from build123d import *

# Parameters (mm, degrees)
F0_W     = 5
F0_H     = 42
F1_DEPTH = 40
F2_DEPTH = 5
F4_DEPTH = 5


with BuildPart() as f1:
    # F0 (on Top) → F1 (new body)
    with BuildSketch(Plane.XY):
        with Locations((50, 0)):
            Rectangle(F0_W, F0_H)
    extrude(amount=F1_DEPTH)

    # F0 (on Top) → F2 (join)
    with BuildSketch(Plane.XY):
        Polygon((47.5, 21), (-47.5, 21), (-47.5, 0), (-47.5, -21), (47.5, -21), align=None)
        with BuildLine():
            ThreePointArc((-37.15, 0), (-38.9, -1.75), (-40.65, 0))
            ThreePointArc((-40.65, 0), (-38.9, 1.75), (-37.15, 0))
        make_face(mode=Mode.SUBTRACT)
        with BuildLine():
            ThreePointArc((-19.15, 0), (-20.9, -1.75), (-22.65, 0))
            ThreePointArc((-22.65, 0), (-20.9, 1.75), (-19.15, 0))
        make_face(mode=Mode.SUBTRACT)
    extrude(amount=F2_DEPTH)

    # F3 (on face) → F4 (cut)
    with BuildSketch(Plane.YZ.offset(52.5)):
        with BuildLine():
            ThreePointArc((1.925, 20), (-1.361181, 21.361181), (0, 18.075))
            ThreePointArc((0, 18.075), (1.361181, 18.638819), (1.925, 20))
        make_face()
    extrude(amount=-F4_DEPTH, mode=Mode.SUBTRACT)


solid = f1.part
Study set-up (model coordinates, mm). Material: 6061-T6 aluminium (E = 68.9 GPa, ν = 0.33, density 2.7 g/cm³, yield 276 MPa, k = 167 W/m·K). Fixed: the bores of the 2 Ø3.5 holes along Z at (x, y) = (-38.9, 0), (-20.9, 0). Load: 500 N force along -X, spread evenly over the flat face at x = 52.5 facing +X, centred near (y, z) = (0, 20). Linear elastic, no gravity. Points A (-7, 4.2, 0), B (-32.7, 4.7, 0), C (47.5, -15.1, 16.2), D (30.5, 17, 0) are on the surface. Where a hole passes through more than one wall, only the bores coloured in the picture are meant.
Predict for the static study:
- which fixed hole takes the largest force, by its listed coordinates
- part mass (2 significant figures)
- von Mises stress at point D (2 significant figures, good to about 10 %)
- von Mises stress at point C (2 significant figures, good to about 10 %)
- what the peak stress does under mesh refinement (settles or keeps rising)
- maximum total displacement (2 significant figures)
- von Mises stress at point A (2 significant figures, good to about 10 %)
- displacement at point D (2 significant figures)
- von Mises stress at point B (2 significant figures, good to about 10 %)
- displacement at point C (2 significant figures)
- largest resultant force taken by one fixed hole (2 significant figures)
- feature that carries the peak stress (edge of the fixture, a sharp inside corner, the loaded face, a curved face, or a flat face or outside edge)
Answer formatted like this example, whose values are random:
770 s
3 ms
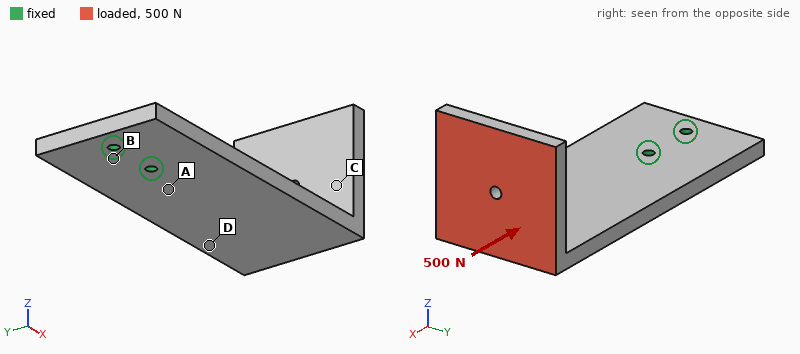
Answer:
(-20.9, 0)
76 g
48 MPa
19 MPa
keeps rising
1.2 mm
44 MPa
0.41 mm
12 MPa
0.77 mm
440 N
edge of the fixture
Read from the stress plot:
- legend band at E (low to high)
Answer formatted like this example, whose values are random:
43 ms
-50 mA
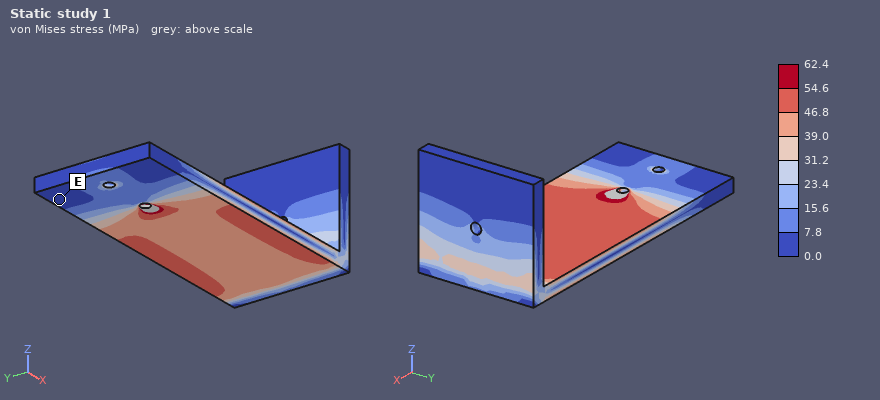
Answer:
0.0 to 7.8 MPa
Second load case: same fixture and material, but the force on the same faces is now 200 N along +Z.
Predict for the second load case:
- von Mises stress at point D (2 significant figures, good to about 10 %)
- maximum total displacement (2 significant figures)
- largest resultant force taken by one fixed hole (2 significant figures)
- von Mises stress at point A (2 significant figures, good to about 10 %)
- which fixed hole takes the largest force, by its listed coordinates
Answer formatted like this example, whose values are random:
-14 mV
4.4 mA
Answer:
26 MPa
1.2 mm
620 N
63 MPa
(-20.9, 0)
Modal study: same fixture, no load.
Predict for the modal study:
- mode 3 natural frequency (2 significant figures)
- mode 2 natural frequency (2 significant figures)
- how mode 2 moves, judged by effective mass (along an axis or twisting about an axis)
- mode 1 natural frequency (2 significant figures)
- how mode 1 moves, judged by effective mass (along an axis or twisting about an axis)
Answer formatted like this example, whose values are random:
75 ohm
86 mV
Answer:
1700 Hz
960 Hz
along Y
410 Hz
along Z
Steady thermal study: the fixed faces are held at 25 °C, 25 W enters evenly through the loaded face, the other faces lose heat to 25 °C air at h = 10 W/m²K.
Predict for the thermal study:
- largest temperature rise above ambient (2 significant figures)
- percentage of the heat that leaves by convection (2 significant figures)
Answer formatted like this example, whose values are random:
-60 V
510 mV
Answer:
61 K
12 %
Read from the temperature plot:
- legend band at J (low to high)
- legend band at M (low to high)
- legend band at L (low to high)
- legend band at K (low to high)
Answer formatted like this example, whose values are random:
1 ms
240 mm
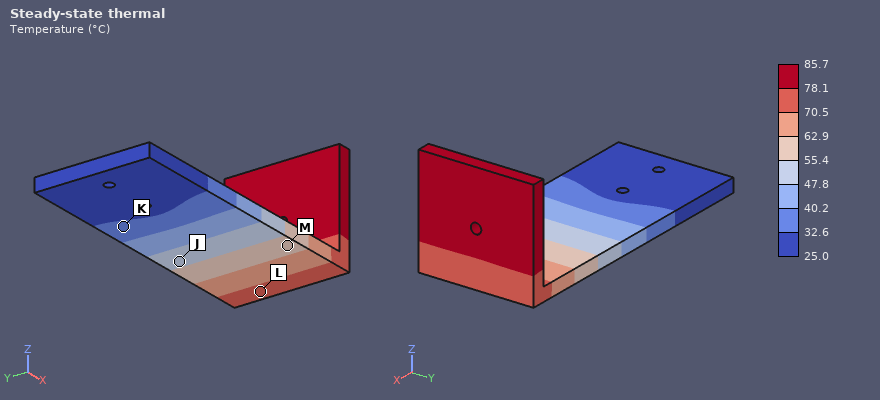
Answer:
47.8 to 55.4 °C
55.4 to 62.9 °C
70.5 to 78.1 °C
32.6 to 40.2 °C
